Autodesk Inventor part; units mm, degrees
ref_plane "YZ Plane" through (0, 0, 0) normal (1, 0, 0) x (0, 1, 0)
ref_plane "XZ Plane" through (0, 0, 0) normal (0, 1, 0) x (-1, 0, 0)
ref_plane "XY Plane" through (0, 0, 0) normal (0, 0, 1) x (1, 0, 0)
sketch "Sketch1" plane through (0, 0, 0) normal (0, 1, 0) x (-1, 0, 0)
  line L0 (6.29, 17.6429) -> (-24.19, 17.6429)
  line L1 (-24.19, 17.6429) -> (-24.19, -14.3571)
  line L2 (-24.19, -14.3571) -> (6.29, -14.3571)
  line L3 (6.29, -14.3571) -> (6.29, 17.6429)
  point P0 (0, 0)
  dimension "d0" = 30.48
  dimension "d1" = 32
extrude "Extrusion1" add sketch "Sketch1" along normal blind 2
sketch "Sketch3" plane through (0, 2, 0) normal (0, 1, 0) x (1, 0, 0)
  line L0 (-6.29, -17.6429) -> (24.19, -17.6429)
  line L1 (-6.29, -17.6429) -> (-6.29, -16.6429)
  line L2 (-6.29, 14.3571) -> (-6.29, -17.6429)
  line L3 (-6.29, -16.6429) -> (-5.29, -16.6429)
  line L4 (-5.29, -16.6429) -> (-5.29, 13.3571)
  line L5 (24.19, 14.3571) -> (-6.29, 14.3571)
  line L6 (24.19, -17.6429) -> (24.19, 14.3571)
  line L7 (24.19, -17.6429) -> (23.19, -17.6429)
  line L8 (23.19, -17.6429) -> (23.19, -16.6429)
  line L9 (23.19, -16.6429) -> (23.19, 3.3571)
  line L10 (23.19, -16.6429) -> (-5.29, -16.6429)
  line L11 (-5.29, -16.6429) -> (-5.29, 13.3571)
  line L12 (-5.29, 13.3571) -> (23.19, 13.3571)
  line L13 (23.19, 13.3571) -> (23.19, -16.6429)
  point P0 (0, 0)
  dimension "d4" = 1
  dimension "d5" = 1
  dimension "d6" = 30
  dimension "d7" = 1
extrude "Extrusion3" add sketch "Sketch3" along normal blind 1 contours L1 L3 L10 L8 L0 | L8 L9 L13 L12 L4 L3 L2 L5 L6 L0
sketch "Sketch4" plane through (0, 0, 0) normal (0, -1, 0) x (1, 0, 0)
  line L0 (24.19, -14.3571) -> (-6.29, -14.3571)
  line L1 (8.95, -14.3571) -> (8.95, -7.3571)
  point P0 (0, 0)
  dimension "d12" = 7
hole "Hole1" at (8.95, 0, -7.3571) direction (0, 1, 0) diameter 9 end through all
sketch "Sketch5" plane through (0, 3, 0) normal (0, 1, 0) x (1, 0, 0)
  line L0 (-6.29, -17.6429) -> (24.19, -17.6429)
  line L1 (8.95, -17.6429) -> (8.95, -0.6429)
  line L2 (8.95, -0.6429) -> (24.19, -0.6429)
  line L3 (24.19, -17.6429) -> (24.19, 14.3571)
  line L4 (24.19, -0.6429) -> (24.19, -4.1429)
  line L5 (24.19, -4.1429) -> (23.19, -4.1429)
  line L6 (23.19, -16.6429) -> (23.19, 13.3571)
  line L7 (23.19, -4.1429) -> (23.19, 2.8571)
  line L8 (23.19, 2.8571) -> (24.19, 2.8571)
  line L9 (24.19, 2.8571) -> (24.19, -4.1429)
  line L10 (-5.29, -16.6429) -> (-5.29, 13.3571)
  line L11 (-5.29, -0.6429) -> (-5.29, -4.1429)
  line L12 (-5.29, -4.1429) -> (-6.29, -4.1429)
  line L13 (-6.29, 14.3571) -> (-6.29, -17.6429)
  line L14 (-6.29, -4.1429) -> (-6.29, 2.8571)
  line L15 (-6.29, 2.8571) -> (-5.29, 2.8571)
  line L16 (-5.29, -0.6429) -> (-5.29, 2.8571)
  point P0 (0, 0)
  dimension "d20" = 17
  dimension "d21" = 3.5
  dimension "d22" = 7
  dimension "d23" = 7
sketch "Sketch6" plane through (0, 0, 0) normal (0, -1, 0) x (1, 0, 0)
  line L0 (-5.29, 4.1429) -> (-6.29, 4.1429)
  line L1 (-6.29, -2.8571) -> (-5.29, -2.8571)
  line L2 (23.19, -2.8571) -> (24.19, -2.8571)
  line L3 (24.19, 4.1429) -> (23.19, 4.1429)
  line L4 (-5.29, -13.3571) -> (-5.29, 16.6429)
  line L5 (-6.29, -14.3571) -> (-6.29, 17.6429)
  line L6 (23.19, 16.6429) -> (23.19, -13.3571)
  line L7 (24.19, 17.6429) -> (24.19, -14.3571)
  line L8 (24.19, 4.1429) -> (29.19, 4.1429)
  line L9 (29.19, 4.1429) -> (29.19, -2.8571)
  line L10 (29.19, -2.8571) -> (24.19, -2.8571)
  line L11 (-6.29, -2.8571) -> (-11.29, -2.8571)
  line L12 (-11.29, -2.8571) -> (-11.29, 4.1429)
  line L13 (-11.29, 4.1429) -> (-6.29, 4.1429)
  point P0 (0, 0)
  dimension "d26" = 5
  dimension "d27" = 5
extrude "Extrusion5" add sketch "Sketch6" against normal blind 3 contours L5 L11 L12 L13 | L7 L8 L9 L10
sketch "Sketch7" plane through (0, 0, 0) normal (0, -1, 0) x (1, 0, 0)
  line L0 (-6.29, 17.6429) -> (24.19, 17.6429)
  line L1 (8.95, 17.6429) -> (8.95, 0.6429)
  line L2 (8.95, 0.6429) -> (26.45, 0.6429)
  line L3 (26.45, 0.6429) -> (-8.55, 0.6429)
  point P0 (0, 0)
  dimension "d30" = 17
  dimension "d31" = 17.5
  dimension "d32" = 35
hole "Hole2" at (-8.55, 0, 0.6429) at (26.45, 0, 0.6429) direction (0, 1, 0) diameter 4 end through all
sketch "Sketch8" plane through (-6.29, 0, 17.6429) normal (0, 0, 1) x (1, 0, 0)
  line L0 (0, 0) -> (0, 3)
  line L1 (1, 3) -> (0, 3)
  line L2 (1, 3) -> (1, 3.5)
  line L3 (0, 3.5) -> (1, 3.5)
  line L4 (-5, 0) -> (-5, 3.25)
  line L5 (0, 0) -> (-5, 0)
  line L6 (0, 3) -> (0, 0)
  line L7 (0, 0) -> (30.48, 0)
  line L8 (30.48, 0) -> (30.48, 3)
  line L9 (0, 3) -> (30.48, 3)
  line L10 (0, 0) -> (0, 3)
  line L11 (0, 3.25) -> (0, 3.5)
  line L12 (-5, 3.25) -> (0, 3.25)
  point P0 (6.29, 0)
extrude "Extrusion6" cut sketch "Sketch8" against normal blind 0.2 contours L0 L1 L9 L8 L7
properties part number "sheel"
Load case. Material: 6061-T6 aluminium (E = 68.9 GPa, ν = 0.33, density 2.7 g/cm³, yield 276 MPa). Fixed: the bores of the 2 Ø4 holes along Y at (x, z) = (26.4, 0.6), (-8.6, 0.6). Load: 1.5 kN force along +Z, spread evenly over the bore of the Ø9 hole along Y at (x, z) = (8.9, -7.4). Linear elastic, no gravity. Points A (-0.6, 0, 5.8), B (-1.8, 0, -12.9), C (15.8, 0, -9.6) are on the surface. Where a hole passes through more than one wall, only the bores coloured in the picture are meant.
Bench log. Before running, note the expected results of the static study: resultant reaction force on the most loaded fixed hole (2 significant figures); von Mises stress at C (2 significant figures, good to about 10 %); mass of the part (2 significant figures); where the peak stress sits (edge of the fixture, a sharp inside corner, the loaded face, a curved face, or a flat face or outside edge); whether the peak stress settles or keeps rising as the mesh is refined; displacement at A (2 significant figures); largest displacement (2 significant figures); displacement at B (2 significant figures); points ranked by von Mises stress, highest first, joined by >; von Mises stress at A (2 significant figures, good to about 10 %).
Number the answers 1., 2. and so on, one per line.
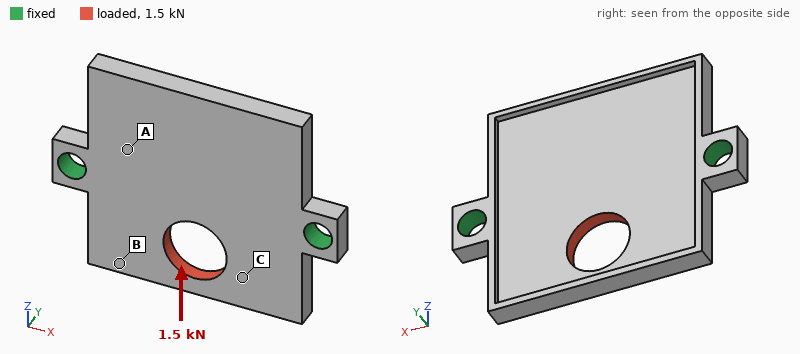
1. 760 N
2. 36 MPa
3. 5.6 g
4. edge of the fixture
5. keeps rising
6. 9.7 µm
7. 23 µm
8. 16 µm
9. C > A > B
10. 23 MPa
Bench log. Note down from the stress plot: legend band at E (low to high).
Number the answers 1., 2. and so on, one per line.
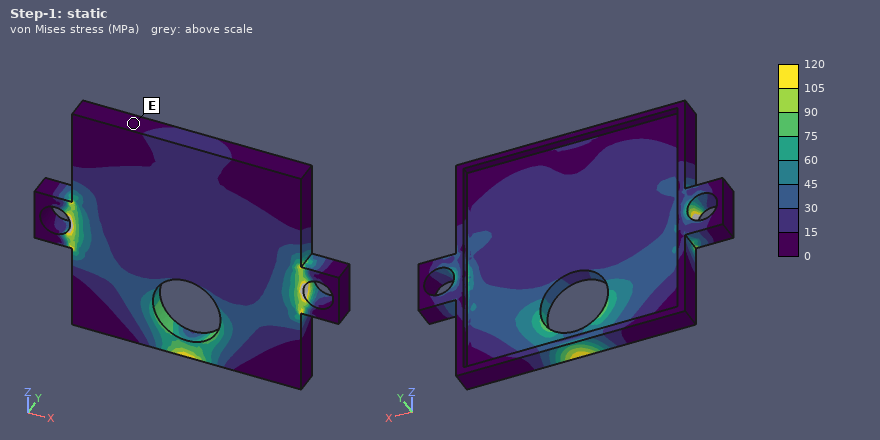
1. 0 to 15 MPa
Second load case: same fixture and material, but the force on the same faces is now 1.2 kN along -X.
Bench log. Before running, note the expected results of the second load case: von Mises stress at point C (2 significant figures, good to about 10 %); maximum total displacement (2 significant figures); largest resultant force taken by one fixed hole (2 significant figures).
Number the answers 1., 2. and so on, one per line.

1. 33 MPa
2. 19 µm
3. 670 N
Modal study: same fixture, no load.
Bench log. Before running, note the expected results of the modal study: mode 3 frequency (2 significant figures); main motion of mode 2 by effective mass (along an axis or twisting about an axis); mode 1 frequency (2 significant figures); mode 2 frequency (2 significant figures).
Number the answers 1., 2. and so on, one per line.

1. 9900 Hz
2. along Y
3. 4600 Hz
4. 6300 Hz
